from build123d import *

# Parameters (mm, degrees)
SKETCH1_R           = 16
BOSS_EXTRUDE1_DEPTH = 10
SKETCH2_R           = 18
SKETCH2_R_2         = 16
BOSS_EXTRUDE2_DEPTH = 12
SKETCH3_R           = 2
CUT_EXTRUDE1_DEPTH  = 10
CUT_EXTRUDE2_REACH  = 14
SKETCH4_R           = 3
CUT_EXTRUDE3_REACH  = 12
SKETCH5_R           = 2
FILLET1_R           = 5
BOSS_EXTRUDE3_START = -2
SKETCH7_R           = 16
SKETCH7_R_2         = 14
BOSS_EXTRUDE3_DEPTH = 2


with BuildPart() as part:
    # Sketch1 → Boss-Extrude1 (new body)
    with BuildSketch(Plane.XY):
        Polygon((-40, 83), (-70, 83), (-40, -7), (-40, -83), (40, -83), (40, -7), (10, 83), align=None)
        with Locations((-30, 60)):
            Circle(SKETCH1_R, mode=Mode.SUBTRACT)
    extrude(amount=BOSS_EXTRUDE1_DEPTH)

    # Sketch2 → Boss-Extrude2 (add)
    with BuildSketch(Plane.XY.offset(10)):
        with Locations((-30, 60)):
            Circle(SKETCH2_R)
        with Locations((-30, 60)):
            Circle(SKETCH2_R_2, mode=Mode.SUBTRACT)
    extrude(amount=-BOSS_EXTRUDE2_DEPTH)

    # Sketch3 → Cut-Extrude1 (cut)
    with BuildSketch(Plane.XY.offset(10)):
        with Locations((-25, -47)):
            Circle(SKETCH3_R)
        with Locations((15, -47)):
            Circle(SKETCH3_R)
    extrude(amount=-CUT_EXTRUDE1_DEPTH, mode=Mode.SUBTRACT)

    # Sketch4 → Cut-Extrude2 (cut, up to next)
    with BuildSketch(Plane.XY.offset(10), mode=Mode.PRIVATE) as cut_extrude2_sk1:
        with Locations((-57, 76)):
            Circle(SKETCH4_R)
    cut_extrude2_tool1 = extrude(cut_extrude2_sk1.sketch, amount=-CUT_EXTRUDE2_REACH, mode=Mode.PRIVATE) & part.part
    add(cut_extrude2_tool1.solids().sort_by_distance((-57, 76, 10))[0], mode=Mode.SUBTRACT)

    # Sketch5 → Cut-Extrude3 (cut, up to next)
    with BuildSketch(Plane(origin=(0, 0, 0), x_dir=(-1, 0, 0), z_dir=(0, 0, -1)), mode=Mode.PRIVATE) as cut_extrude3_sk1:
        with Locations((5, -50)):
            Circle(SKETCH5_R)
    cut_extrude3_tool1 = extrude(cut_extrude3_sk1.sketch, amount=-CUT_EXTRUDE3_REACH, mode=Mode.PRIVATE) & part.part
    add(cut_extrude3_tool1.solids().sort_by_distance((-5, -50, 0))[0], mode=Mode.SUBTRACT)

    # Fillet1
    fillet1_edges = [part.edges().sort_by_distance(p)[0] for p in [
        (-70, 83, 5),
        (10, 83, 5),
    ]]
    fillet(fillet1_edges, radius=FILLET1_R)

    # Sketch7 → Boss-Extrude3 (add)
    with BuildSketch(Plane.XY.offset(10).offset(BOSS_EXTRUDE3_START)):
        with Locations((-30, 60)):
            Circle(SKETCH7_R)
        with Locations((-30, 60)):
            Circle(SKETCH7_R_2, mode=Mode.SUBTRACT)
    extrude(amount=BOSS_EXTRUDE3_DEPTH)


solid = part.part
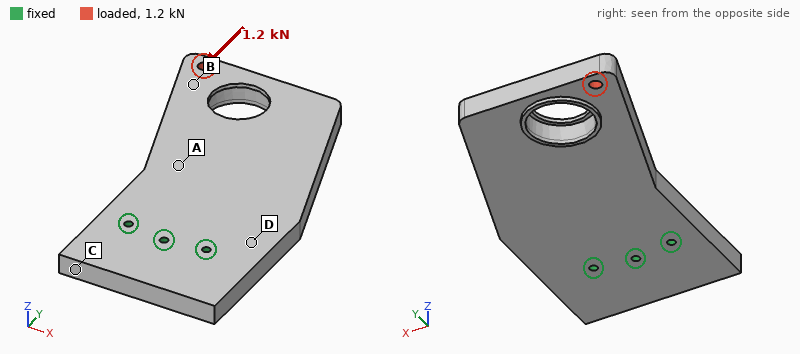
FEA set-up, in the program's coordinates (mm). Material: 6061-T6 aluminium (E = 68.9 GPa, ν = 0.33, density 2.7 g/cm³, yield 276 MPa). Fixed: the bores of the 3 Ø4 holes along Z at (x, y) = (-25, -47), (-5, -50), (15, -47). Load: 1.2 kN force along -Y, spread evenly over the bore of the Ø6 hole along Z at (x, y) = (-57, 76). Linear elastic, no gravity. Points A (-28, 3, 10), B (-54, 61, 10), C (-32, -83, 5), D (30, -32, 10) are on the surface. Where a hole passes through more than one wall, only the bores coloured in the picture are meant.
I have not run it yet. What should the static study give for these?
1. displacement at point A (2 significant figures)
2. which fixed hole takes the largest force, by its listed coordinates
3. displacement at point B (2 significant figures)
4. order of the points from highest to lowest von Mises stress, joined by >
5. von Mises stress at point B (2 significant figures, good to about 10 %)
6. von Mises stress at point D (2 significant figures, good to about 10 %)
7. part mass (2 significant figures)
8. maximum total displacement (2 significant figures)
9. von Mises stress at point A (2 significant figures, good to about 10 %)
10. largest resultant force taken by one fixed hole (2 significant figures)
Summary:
8.0 µm
(-25, -47)
30 µm
B > A > D > C
6.9 MPa
2.7 MPa
340 g
38 µm
5.1 MPa
1.9 kN
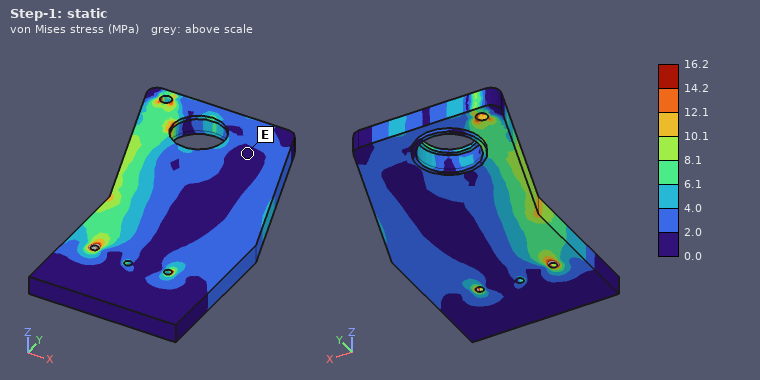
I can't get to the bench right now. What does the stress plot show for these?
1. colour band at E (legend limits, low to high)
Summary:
0.0 to 2.0 MPa
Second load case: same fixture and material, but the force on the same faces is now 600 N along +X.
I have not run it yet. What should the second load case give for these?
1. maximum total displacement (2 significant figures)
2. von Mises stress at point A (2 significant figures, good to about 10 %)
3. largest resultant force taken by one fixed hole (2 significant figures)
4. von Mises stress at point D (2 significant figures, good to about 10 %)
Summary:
38 µm
2.9 MPa
1.8 kN
3.4 MPa
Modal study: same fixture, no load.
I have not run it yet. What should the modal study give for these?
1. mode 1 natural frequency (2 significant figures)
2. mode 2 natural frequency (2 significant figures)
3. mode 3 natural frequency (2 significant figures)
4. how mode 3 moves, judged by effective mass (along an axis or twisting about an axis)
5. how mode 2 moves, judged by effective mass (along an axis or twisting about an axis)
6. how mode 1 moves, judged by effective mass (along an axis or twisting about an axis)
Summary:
500 Hz
1500 Hz
2500 Hz
along X
twisting about Y
along Z
